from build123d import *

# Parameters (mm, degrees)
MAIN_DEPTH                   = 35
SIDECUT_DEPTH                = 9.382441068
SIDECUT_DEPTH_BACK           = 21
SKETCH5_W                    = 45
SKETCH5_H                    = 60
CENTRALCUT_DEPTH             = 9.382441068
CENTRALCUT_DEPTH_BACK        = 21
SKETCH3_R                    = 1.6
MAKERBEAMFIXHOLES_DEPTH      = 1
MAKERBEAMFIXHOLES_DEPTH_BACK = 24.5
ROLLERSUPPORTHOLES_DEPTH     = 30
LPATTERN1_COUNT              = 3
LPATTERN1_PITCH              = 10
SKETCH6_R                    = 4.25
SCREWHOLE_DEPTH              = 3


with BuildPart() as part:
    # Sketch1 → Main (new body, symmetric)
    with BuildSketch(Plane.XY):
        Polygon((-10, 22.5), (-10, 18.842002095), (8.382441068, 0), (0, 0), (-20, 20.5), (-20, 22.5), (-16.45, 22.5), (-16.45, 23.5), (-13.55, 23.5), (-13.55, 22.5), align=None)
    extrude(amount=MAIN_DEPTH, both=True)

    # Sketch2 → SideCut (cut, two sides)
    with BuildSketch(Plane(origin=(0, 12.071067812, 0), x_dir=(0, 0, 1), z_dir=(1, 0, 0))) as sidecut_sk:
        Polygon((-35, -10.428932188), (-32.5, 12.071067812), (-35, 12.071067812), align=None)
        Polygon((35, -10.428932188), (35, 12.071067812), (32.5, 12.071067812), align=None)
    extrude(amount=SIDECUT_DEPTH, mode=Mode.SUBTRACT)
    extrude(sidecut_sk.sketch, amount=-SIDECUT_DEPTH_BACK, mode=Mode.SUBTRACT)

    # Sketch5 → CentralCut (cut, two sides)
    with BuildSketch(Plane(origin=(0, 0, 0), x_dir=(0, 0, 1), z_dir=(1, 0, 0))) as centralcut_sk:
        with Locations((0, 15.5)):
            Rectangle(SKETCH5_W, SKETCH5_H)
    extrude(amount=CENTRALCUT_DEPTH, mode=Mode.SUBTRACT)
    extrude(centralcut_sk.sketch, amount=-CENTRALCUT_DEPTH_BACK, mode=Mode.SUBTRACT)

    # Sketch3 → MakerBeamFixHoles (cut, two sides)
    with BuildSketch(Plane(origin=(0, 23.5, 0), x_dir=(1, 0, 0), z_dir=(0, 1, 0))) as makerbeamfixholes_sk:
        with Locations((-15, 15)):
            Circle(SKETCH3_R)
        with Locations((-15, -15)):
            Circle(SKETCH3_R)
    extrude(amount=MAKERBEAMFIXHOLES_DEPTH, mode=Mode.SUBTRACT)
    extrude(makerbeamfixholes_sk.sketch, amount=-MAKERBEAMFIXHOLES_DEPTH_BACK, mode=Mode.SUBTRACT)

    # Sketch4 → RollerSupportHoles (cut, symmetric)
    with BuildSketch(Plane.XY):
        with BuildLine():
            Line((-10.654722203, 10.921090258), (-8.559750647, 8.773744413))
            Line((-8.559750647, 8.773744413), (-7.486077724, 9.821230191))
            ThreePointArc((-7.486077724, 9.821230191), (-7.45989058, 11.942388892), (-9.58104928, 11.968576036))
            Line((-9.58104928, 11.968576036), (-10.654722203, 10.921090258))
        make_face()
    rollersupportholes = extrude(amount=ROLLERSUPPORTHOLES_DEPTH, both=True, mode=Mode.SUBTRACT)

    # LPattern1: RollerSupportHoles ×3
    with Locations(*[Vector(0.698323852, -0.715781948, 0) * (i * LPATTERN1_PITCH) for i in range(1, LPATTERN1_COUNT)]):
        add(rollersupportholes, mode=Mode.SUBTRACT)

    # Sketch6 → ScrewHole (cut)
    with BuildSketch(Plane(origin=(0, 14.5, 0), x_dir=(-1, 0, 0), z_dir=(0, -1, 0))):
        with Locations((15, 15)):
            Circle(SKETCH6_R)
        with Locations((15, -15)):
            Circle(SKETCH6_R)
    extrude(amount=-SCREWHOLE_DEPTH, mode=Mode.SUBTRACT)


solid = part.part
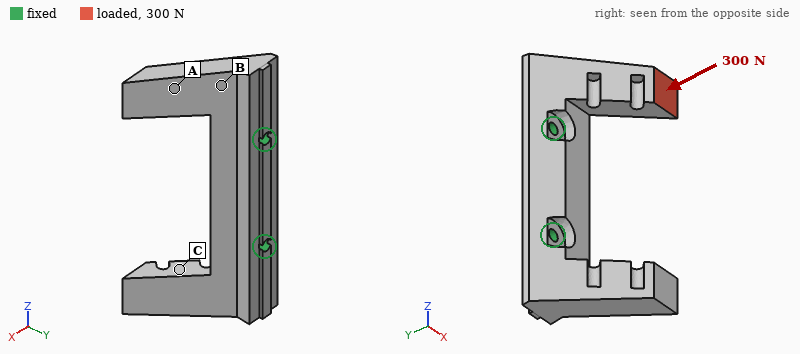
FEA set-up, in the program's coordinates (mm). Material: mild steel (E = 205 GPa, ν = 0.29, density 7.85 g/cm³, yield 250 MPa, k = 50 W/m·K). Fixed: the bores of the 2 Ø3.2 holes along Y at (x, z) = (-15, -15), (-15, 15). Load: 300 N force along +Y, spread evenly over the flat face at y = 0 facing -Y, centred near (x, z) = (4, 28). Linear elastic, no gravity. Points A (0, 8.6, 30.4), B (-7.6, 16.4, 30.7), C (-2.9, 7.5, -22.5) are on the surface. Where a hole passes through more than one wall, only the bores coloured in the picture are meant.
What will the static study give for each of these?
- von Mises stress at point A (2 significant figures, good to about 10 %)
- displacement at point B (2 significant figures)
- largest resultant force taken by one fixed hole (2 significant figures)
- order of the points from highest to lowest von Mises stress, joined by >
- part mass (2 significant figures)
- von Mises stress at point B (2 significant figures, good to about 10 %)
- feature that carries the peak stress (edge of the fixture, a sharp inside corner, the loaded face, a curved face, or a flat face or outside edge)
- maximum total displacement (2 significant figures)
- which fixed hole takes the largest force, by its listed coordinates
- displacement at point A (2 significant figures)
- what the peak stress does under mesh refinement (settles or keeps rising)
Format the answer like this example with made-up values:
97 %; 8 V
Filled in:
46 MPa; 0.023 mm; 360 N; B > A > C; 57 g; 76 MPa; edge of the fixture; 0.10 mm; (-15, 15); 0.054 mm; keeps rising
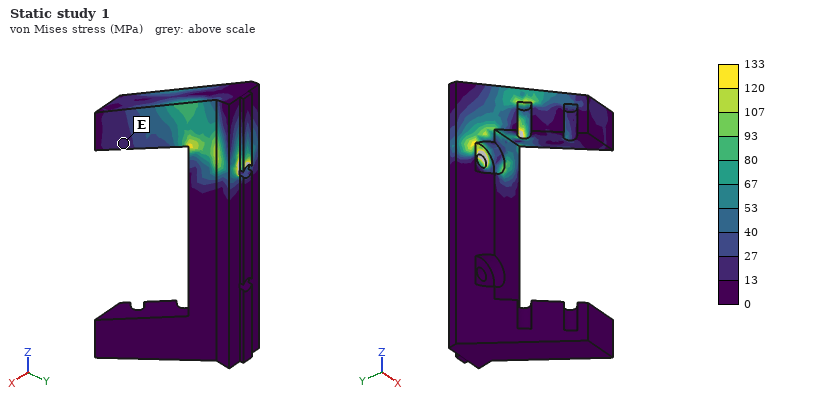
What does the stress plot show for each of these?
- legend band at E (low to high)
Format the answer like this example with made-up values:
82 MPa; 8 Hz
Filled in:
13 to 27 MPa
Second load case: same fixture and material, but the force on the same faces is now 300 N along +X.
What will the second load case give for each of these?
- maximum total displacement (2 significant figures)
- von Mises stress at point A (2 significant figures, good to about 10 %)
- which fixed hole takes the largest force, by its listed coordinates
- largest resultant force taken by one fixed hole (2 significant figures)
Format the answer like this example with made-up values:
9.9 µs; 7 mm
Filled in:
0.11 mm; 48 MPa; (-15, 15); 370 N
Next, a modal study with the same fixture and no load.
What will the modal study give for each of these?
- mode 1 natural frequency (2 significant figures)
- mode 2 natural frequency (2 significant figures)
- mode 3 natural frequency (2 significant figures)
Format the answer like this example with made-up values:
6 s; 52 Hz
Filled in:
3900 Hz; 3900 Hz; 6700 Hz
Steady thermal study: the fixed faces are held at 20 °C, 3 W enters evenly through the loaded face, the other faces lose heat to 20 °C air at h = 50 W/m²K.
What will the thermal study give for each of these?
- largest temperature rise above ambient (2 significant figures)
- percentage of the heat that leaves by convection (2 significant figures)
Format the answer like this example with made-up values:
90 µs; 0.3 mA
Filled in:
32 K; 31 %
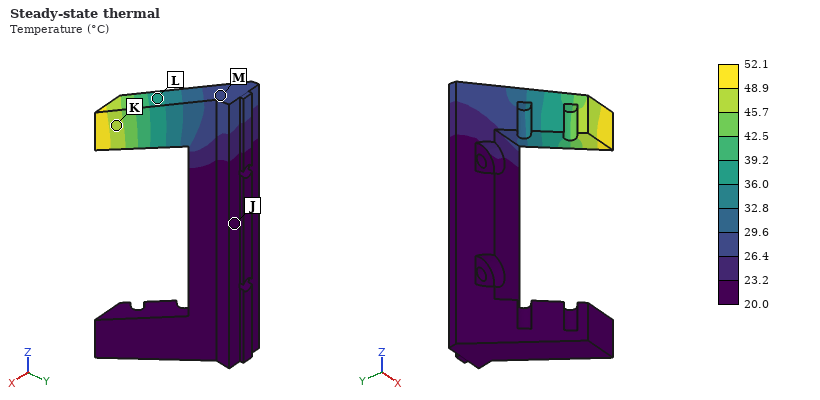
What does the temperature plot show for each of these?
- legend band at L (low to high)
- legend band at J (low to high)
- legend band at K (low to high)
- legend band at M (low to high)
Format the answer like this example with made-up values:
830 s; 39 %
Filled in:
36.0 to 39.2 °C; 20.0 to 23.2 °C; 45.7 to 48.9 °C; 26.4 to 29.6 °C
